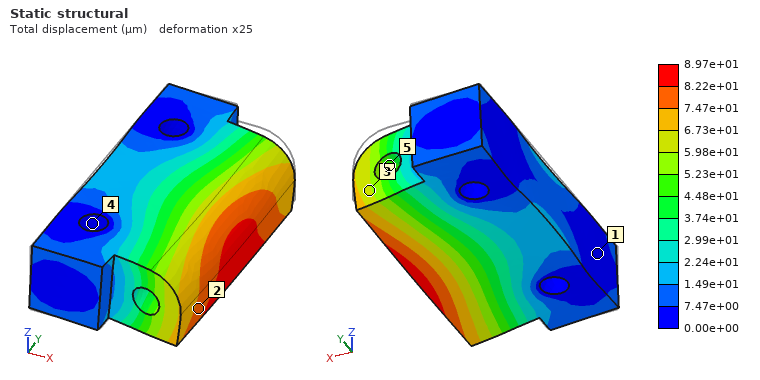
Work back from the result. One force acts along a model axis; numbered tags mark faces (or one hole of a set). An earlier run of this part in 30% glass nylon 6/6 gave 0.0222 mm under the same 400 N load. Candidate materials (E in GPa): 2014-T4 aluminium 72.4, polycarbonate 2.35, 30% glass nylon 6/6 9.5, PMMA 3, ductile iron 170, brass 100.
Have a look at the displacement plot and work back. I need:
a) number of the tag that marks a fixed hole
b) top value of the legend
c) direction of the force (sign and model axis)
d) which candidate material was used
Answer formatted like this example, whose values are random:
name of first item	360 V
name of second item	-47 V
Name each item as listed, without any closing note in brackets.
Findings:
number of the tag that marks a fixed hole	4
top value of the legend	8.97e+01 µm
direction of the force	-Z
which candidate material was used	polycarbonate
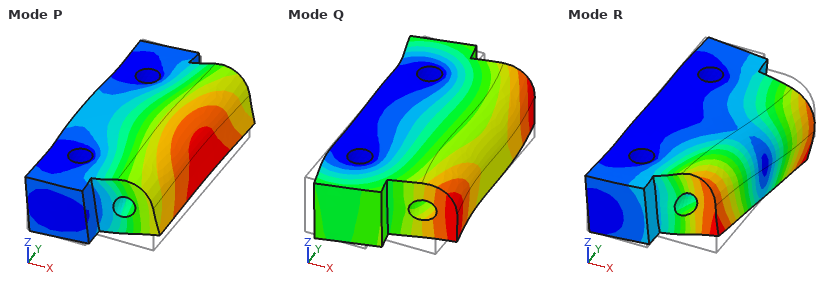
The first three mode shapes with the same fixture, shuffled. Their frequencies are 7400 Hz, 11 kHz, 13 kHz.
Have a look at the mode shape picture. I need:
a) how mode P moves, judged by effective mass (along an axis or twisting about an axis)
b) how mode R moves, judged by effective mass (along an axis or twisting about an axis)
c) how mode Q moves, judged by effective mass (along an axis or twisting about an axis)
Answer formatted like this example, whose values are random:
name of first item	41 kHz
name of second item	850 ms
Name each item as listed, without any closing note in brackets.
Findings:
how mode P moves, judged by effective mass	along Z
how mode R moves, judged by effective mass	twisting about X
how mode Q moves, judged by effective mass	along Y
